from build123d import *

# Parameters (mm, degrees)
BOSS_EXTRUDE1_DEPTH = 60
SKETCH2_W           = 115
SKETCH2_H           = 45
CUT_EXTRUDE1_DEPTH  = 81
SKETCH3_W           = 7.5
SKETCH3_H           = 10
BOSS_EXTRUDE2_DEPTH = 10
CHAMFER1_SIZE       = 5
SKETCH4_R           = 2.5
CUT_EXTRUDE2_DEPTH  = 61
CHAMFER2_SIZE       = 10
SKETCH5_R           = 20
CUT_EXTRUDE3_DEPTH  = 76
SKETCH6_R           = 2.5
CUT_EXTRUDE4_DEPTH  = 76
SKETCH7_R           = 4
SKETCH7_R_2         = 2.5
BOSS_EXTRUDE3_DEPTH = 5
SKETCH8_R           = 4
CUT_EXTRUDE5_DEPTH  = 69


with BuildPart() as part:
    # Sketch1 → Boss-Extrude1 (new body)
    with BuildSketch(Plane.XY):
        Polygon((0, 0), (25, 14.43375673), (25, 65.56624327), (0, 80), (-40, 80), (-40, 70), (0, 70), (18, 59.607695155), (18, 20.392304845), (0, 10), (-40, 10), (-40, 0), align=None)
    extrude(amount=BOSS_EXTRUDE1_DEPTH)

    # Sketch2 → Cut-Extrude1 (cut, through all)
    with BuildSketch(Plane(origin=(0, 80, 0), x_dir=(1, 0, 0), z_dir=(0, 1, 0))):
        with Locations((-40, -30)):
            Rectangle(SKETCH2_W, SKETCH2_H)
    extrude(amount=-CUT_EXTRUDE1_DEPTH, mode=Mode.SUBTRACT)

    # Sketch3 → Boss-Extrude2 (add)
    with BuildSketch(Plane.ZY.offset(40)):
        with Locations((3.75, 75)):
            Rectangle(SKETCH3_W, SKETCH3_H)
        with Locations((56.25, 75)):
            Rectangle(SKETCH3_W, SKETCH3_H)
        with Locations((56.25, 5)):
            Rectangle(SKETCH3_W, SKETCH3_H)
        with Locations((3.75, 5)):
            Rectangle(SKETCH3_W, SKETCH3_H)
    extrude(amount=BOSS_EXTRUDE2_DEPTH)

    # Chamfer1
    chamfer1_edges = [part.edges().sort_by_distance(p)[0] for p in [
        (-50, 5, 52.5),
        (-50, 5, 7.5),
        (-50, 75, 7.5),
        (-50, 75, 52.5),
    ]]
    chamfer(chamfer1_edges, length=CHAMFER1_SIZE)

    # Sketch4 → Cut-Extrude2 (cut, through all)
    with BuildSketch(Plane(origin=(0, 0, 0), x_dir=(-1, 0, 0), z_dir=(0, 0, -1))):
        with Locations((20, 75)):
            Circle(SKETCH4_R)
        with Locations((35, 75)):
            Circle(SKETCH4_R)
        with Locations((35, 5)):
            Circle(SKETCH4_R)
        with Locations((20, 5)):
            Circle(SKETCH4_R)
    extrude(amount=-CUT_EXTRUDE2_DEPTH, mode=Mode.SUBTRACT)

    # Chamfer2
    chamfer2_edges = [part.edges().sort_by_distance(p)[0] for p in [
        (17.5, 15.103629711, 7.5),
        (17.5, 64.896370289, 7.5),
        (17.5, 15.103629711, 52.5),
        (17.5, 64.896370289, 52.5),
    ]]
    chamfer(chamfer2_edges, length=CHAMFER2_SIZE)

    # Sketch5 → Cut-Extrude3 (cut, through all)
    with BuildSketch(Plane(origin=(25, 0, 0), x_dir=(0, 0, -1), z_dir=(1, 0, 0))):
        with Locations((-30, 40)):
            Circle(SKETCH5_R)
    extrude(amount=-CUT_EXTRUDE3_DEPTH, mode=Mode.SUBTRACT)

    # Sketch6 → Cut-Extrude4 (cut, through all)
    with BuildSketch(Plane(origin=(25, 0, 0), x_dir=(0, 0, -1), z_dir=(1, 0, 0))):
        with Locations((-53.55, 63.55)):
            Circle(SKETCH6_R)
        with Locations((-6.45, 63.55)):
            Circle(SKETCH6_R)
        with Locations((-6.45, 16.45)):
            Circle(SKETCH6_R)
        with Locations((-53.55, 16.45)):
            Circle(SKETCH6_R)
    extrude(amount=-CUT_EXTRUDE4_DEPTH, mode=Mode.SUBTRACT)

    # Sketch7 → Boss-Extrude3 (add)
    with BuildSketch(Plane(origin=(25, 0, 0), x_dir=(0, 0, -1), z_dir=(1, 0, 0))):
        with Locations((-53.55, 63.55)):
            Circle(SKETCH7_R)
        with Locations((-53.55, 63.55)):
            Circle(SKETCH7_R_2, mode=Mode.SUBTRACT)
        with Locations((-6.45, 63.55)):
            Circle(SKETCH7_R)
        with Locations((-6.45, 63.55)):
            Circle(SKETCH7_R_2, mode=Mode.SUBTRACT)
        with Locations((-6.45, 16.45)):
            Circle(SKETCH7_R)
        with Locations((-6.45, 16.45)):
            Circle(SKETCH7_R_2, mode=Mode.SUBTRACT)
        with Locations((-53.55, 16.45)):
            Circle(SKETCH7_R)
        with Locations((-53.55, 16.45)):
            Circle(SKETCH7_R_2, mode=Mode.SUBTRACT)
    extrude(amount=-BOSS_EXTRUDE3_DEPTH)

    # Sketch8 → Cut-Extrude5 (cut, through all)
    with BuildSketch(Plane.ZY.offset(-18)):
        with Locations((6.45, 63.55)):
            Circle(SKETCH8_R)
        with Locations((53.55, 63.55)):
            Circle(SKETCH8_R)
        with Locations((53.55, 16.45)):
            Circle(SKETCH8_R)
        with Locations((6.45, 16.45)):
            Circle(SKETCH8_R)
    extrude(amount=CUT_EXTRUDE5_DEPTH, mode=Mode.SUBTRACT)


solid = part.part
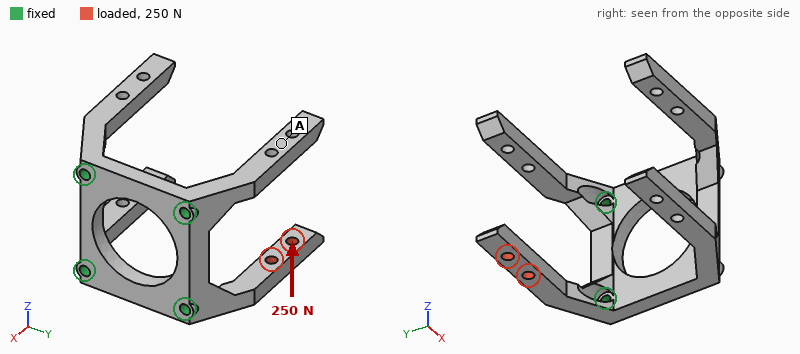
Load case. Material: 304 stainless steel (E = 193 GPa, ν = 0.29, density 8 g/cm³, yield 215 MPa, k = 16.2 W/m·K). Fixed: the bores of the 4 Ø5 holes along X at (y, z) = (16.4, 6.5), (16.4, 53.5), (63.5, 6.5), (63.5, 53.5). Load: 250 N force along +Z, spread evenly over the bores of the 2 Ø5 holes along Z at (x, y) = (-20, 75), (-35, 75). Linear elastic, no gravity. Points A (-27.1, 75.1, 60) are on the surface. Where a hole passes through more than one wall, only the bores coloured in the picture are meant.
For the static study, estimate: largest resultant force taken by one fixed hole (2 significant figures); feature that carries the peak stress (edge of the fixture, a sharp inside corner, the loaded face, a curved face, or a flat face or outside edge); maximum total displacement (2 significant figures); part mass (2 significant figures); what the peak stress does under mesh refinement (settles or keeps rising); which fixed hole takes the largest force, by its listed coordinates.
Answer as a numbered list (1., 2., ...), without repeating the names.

1. 170 N
2. a sharp inside corner
3. 0.23 mm
4. 270 g
5. keeps rising
6. (63.5, 6.5)
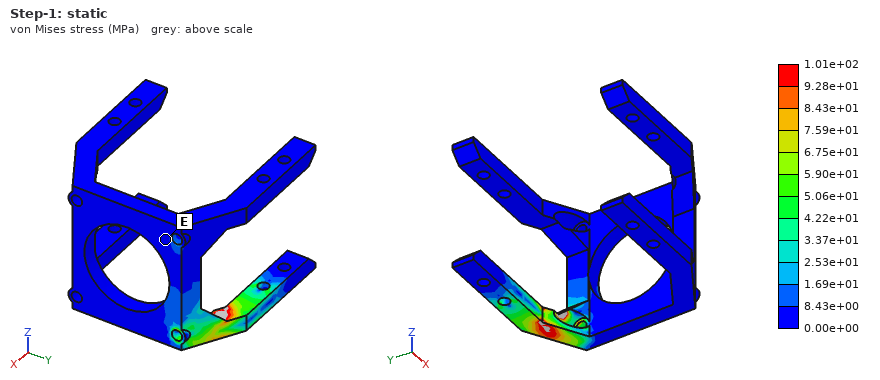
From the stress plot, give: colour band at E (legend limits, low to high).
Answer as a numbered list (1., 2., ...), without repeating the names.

1. 0.00e+00 to 8.43e+00 MPa
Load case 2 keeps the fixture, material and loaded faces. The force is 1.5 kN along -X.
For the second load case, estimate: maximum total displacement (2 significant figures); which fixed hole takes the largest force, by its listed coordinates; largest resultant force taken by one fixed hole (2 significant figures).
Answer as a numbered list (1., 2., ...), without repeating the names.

1. 0.21 mm
2. (63.5, 6.5)
3. 1.6 kN
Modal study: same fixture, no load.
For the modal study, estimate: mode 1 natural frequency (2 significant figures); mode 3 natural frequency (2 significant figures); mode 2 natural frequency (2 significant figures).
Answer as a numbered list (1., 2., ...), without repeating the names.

1. 1200 Hz
2. 1200 Hz
3. 1200 Hz
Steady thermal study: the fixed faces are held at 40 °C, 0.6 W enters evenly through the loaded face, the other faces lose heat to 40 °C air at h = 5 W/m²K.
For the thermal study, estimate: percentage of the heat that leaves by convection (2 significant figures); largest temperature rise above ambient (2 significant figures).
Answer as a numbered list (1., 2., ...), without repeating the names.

1. 28 %
2. 22 K
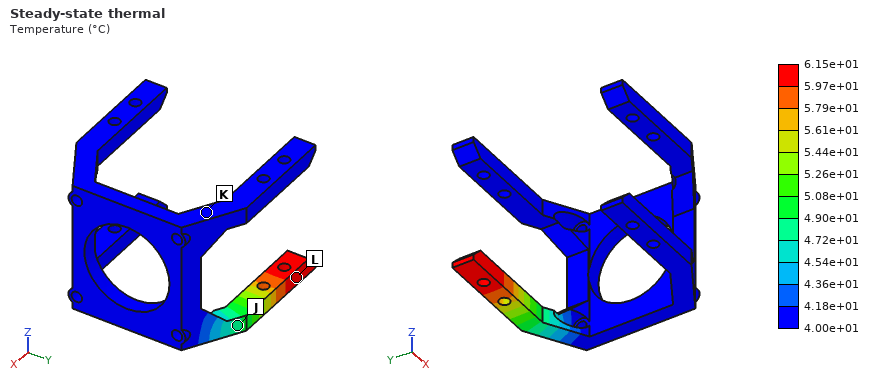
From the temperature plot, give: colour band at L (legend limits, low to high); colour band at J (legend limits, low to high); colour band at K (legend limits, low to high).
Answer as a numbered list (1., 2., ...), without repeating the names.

1. 5.97e+01 to 6.15e+01 °C
2. 4.72e+01 to 4.90e+01 °C
3. 4.00e+01 to 4.18e+01 °C
